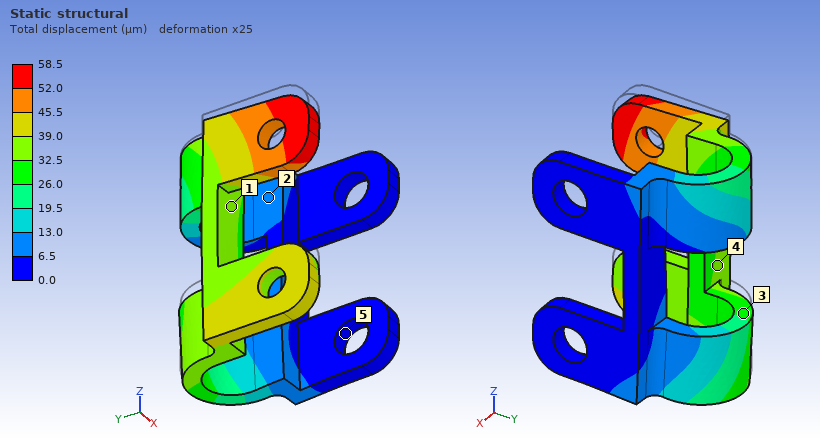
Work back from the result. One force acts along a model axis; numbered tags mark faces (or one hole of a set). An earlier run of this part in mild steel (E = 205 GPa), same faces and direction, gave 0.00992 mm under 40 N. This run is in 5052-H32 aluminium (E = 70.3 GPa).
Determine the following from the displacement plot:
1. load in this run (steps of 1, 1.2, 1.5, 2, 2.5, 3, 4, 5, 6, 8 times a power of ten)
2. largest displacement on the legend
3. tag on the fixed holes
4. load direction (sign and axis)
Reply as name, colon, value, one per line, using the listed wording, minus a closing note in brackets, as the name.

load in this run: 80 N
largest displacement on the legend: 58.5 µm
tag on the fixed holes: 5
load direction: -Z
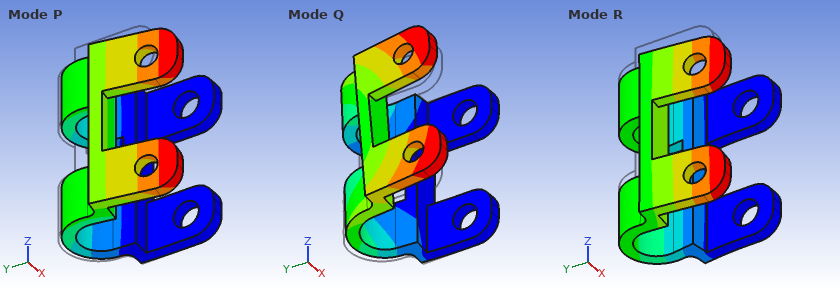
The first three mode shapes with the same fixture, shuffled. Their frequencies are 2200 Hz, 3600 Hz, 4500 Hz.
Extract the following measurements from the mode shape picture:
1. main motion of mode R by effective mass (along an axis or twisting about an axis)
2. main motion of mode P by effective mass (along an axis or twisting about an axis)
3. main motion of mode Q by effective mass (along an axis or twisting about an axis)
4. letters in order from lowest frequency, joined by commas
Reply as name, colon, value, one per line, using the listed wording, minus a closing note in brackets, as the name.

main motion of mode R by effective mass: along X
main motion of mode P by effective mass: along Y
main motion of mode Q by effective mass: along Z
letters in order from lowest frequency, joined by commas: P, Q, R
